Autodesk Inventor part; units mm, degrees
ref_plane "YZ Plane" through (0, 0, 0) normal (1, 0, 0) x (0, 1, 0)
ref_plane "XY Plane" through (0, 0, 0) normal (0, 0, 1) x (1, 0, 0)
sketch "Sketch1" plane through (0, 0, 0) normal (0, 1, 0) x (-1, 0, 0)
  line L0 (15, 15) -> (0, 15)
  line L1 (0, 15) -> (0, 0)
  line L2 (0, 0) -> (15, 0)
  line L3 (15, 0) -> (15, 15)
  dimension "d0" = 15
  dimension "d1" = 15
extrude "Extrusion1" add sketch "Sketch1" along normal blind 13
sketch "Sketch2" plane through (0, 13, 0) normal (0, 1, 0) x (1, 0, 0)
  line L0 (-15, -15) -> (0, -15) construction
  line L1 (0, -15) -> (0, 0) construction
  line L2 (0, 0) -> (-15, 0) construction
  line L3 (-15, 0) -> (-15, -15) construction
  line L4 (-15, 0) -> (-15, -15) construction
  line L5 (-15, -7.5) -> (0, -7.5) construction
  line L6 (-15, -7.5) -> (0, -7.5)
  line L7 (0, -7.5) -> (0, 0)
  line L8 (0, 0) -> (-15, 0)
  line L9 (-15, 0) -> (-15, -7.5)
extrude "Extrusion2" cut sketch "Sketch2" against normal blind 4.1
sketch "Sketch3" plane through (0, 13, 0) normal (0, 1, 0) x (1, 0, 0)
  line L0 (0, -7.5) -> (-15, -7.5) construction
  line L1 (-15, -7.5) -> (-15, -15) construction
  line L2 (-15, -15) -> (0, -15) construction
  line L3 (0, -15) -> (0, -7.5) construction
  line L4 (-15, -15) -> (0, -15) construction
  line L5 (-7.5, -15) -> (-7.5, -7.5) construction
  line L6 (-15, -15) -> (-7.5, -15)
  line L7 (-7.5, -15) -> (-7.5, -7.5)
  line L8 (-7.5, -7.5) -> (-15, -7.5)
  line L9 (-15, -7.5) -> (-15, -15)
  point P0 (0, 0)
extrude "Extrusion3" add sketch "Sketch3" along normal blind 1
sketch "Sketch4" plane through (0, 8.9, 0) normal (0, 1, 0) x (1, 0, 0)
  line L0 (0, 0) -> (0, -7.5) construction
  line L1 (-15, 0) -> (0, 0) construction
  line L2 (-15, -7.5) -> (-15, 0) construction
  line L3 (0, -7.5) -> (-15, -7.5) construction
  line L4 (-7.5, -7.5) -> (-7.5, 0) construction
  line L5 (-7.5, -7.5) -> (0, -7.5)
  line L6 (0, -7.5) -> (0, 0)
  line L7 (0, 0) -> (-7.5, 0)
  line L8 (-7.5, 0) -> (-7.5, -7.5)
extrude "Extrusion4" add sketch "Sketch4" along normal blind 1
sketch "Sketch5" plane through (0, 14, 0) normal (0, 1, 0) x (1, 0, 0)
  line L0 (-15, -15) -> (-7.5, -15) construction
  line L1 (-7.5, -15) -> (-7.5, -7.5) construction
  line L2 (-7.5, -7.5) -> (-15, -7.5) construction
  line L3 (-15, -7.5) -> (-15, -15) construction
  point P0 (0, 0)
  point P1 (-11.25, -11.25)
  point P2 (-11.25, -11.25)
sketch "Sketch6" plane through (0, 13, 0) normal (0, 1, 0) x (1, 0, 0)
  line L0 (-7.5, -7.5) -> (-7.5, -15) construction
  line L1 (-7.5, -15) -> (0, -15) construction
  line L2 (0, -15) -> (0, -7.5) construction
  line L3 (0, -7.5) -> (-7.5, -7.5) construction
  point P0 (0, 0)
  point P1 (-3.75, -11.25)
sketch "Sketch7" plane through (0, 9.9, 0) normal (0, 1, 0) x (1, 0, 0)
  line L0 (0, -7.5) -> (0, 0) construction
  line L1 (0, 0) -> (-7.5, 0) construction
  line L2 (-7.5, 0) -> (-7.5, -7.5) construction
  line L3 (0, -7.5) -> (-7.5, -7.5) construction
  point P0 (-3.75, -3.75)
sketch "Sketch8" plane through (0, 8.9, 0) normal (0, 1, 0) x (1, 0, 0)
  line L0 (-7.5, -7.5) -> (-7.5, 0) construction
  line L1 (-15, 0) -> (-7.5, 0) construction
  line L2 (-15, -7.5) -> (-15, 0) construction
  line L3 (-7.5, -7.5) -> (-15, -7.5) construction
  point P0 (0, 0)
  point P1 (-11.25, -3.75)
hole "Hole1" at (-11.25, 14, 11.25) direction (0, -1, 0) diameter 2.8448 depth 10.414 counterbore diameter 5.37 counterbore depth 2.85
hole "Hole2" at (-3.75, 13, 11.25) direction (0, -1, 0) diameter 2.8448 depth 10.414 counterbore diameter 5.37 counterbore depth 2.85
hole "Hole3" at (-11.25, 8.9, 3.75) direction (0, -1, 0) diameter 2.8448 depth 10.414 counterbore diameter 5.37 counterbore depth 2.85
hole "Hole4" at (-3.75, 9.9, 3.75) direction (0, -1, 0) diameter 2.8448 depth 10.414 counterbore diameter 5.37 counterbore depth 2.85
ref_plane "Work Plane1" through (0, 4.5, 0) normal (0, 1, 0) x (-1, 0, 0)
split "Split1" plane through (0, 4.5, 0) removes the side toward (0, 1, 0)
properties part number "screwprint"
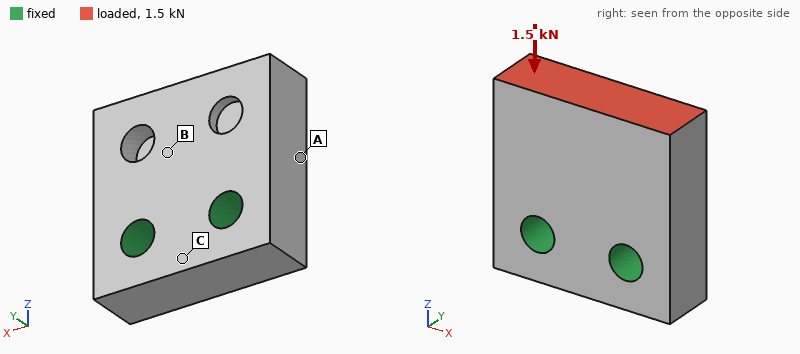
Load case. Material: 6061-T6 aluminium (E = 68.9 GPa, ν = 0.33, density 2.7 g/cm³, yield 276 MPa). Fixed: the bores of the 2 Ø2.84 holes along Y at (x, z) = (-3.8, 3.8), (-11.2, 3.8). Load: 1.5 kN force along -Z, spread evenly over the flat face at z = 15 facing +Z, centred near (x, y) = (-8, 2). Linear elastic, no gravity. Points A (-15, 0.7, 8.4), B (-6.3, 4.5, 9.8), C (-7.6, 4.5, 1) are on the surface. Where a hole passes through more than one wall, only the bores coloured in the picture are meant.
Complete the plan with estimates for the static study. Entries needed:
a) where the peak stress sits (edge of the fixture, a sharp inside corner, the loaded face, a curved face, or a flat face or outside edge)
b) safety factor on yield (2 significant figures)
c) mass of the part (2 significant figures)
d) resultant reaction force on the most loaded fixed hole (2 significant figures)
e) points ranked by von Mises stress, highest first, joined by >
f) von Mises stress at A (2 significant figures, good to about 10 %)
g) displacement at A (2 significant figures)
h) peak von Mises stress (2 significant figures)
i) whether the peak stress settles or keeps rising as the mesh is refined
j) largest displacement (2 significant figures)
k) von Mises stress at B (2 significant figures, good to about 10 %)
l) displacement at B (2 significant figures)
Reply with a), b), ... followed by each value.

a) a curved face
b) 4.1
c) 2.5 g
d) 760 N
e) B > A > C
f) 16 MPa
g) 1.9 µm
h) 68 MPa
i) settles
j) 5.0 µm
k) 31 MPa
l) 2.1 µm
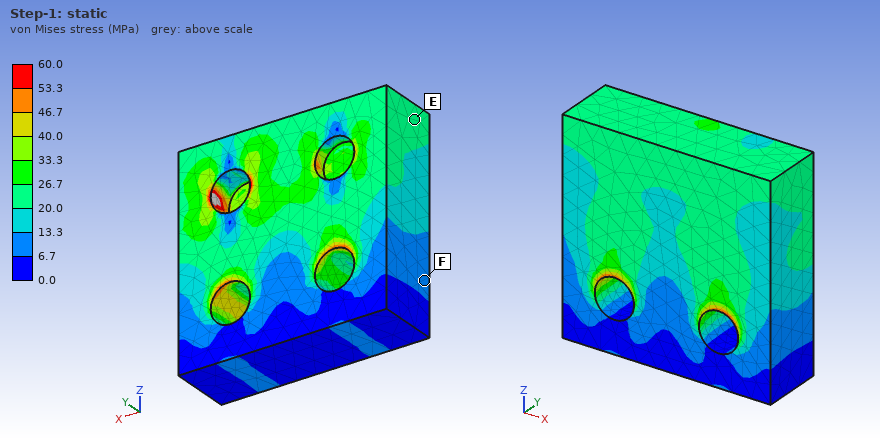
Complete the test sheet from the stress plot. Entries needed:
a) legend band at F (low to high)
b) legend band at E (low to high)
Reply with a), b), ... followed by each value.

a) 6.7 to 13.3 MPa
b) 20.0 to 26.7 MPa
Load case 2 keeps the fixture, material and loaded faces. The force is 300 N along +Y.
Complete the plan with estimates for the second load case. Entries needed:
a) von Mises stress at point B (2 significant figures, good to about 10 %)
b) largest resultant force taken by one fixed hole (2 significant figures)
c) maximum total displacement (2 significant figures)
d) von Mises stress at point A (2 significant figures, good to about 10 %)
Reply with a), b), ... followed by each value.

a) 36 MPa
b) 150 N
c) 19 µm
d) 23 MPa
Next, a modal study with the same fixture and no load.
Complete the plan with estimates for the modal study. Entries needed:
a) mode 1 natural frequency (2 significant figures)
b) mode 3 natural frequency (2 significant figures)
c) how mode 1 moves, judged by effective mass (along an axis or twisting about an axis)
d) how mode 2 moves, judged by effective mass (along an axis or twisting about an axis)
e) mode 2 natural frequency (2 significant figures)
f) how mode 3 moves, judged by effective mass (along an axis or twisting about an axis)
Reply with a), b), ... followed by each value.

a) 29 kHz
b) 51 kHz
c) along Y
d) twisting about Z
e) 45 kHz
f) along X
